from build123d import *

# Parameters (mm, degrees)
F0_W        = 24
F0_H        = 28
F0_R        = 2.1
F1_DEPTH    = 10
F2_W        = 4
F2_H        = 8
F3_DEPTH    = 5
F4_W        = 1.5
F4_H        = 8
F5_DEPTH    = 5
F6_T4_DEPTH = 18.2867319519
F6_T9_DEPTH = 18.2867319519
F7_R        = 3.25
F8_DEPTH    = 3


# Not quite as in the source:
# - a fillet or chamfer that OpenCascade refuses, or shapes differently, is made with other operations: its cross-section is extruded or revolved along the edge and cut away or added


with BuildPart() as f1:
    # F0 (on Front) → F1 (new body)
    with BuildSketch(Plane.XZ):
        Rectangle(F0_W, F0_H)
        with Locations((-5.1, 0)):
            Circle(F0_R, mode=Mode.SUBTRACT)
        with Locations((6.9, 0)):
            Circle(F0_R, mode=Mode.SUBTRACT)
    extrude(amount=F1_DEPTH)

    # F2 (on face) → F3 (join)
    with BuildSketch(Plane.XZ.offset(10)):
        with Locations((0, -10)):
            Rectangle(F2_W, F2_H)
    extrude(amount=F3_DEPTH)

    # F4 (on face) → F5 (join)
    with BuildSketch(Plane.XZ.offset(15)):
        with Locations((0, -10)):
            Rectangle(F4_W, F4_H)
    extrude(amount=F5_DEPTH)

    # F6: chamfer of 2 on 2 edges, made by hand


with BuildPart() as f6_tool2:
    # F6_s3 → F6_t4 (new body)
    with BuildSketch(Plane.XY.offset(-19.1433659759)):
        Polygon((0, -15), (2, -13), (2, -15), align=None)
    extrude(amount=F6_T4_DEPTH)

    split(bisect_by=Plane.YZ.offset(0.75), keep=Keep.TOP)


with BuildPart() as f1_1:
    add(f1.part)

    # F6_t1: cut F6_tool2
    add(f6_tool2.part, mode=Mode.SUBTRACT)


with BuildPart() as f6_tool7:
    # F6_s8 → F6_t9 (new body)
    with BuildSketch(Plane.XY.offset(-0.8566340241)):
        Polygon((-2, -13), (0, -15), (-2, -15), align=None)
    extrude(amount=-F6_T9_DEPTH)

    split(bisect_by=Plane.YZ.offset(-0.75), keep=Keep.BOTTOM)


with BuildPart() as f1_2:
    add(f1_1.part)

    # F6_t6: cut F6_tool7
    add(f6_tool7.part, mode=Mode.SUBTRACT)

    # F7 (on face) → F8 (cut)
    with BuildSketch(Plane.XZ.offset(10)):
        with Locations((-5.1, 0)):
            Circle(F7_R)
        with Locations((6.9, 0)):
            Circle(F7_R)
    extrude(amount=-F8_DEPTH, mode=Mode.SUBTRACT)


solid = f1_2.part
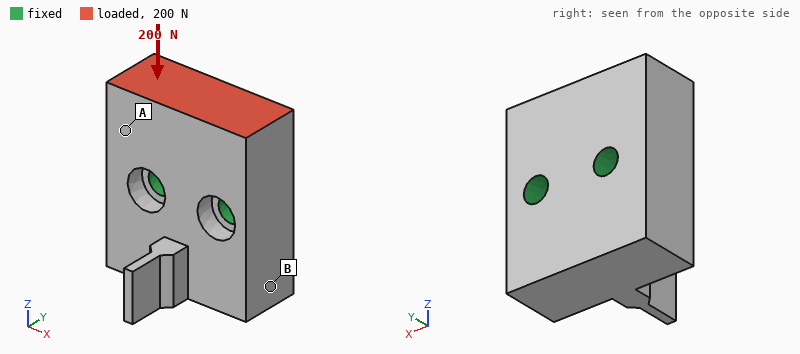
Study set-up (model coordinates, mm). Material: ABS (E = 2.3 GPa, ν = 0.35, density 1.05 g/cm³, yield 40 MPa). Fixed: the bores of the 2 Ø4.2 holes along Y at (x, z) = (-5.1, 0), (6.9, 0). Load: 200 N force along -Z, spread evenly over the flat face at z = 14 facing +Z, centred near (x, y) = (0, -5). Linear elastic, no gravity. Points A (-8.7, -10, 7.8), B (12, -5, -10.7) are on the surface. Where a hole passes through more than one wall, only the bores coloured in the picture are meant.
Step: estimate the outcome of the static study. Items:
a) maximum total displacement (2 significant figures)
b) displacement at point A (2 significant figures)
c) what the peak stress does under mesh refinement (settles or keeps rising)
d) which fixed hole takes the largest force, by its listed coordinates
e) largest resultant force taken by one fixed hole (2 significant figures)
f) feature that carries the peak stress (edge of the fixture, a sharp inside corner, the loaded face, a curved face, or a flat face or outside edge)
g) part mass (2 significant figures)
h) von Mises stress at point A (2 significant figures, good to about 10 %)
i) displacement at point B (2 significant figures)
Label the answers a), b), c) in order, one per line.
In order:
a) 12 µm
b) 8.1 µm
c) keeps rising
d) (-5.1, 0)
e) 110 N
f) edge of the fixture
g) 6.8 g
h) 0.76 MPa
i) 2.6 µm
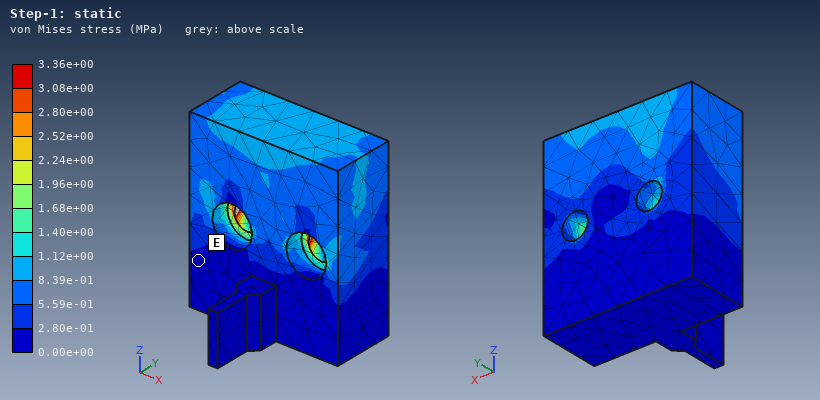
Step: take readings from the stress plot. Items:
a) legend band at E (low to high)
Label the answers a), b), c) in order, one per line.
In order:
a) 0.00e+00 to 2.80e-01 MPa
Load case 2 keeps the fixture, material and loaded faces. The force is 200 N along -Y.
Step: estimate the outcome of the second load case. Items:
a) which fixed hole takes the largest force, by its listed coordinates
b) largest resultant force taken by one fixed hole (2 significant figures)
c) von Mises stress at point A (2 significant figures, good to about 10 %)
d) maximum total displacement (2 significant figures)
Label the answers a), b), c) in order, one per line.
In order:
a) (-5.1, 0)
b) 110 N
c) 2.8 MPa
d) 92 µm
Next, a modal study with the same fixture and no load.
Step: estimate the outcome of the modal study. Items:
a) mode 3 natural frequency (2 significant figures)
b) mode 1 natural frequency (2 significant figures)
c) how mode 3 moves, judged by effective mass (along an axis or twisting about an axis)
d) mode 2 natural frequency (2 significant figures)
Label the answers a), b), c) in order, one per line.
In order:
a) 8600 Hz
b) 6100 Hz
c) along Y
d) 7400 Hz
